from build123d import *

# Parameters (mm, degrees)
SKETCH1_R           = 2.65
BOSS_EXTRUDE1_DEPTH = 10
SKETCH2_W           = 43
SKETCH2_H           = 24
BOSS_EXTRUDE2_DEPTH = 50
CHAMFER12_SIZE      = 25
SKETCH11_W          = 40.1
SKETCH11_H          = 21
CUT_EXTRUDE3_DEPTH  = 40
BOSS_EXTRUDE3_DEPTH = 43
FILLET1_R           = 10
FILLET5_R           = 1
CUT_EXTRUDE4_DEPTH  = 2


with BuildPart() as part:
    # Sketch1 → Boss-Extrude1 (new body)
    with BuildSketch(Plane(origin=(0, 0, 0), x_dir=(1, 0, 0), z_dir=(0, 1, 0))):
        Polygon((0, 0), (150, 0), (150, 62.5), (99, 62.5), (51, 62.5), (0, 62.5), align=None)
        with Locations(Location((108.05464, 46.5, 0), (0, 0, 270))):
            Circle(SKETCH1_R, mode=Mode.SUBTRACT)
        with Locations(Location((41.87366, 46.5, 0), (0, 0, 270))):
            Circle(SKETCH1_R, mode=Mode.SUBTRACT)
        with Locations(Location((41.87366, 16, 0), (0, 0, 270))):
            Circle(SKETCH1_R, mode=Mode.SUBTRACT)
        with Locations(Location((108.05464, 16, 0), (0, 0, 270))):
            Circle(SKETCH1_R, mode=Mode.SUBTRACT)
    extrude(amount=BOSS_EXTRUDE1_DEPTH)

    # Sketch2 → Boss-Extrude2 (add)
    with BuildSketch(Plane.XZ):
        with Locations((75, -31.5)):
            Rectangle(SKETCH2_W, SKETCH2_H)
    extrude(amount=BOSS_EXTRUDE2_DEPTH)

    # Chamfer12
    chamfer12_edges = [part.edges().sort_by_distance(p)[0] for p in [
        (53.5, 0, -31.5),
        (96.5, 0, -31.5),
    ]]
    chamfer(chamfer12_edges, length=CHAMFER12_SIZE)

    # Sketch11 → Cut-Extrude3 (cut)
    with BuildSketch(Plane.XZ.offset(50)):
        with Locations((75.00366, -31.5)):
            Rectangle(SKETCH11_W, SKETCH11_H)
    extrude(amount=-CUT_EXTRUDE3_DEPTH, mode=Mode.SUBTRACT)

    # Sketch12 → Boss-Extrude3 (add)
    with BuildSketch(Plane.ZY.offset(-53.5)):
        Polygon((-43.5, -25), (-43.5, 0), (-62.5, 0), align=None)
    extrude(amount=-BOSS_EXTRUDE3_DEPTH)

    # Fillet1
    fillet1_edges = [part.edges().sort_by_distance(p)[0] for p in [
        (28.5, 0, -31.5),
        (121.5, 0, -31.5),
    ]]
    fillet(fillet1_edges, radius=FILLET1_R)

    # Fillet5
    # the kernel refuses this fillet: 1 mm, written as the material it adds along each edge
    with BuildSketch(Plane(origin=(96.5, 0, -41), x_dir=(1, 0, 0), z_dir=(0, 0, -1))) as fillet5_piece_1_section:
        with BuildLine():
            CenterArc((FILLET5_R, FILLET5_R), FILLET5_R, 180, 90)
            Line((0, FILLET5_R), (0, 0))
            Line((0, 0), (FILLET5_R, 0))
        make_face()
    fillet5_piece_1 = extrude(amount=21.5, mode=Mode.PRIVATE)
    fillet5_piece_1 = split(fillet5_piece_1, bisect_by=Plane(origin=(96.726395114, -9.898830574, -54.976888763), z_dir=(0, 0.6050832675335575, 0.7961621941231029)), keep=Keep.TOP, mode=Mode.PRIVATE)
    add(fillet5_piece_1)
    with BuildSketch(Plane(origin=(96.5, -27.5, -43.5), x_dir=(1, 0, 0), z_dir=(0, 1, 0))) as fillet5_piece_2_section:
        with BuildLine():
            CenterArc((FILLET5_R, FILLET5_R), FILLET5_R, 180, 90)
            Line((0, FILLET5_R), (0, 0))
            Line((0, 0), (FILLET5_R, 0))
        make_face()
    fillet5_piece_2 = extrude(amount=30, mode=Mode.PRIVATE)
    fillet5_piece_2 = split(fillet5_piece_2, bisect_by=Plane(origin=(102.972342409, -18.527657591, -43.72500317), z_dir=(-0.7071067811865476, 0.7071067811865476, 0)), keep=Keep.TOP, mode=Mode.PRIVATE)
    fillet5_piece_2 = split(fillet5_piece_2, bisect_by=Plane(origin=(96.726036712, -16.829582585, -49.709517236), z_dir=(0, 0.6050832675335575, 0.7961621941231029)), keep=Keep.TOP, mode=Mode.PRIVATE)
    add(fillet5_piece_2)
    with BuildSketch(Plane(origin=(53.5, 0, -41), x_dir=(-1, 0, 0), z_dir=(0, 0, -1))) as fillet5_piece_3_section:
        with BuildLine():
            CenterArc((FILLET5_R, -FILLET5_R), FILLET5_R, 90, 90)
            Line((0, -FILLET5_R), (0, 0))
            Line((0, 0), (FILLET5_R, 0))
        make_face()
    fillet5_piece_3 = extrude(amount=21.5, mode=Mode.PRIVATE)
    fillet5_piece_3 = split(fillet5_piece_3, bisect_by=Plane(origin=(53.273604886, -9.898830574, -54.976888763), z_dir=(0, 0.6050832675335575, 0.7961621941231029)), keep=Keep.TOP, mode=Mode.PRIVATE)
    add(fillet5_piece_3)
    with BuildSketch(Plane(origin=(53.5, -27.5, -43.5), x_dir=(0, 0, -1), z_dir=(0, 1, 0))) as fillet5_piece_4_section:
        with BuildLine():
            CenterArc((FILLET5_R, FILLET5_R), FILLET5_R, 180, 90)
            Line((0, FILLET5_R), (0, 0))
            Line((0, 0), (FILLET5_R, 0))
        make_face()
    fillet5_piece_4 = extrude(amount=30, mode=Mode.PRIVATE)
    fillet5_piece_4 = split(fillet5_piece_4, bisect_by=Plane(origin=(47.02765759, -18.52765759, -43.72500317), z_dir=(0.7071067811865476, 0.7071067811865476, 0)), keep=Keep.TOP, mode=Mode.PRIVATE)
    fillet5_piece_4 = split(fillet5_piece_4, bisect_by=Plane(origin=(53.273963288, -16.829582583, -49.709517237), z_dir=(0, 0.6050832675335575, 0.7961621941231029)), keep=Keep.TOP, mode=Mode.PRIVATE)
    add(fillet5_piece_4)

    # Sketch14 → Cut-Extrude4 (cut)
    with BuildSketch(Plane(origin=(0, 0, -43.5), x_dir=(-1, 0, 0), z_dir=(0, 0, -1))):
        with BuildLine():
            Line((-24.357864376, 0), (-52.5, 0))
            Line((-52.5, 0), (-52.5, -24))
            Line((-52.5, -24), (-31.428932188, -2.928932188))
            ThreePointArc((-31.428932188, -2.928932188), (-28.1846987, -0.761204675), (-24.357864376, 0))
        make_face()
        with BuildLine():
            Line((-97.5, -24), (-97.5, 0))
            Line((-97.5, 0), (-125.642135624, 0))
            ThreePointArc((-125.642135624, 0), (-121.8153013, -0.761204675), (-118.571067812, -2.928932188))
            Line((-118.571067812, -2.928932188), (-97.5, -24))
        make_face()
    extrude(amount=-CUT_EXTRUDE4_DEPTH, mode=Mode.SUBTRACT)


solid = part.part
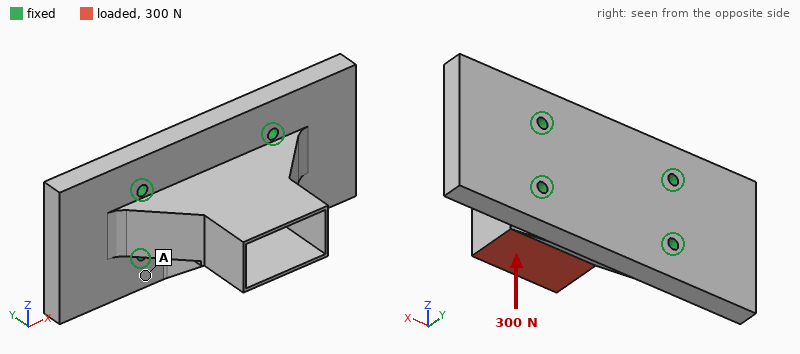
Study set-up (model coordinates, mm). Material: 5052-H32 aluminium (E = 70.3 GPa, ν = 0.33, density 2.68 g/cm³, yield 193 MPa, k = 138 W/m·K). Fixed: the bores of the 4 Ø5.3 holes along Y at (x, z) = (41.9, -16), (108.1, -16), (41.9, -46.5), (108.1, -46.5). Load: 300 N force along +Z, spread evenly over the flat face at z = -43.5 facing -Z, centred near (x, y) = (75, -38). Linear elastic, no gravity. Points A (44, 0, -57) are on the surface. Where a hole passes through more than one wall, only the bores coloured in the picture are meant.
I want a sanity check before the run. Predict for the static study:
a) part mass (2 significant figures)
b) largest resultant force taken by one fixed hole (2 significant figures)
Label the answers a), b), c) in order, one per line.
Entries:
a) 360 g
b) 220 N
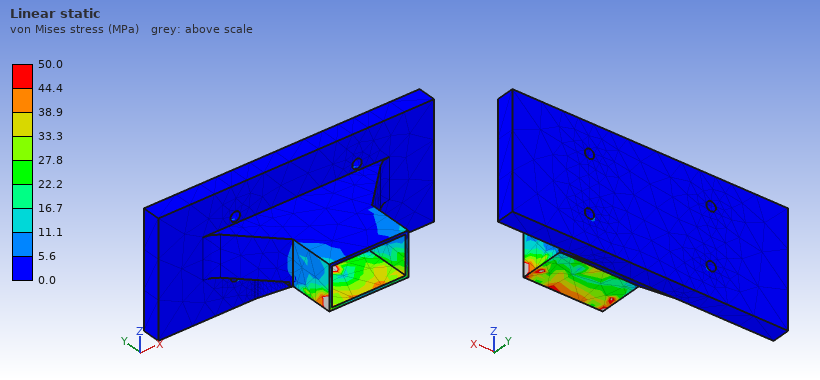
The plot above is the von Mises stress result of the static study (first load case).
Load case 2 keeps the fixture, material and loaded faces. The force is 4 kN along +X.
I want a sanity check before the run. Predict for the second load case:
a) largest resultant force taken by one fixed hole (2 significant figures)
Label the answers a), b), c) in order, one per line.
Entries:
a) 2.2 kN
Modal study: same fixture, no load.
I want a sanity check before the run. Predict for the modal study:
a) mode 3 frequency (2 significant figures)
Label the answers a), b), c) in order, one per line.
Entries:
a) 5100 Hz
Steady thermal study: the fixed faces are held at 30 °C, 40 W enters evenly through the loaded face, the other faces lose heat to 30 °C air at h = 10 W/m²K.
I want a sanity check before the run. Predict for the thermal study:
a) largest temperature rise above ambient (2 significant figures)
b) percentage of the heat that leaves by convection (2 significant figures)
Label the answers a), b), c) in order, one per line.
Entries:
a) 56 K
b) 4.9 %
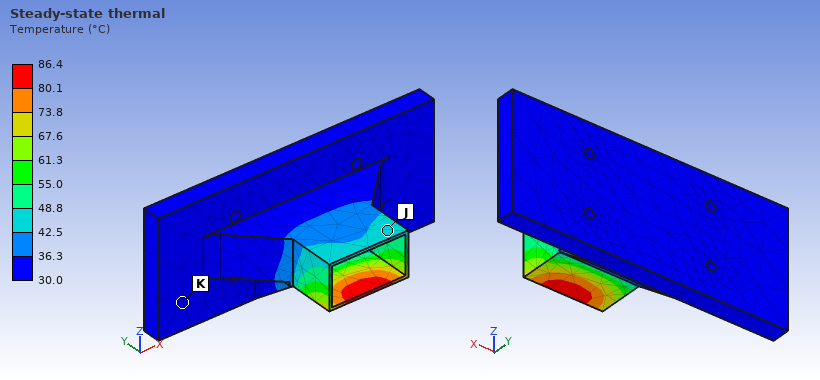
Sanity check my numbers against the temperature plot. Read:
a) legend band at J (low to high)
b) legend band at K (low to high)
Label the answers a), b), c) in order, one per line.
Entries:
a) 42.5 to 48.8 °C
b) 30.0 to 36.3 °C
